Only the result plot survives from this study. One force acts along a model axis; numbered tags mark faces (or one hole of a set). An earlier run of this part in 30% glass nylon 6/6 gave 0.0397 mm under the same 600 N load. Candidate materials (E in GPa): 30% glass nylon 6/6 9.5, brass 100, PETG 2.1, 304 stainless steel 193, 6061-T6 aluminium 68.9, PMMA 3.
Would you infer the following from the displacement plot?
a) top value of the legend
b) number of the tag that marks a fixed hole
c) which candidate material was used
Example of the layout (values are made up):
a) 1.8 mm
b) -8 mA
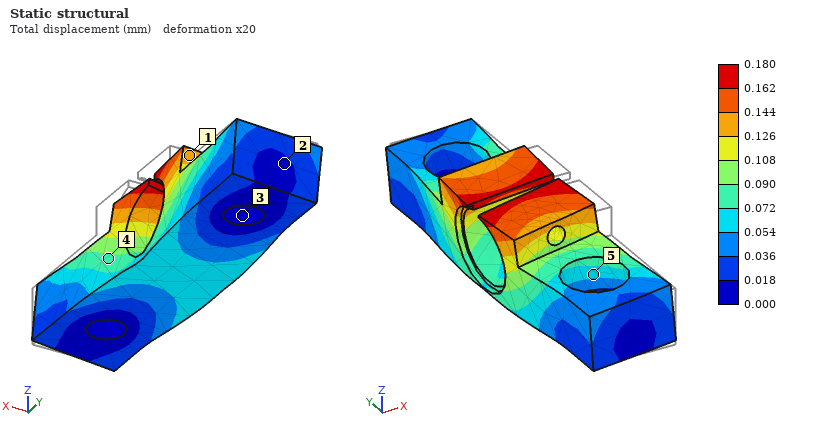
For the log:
a) 0.180 mm
b) 3
c) PETG
